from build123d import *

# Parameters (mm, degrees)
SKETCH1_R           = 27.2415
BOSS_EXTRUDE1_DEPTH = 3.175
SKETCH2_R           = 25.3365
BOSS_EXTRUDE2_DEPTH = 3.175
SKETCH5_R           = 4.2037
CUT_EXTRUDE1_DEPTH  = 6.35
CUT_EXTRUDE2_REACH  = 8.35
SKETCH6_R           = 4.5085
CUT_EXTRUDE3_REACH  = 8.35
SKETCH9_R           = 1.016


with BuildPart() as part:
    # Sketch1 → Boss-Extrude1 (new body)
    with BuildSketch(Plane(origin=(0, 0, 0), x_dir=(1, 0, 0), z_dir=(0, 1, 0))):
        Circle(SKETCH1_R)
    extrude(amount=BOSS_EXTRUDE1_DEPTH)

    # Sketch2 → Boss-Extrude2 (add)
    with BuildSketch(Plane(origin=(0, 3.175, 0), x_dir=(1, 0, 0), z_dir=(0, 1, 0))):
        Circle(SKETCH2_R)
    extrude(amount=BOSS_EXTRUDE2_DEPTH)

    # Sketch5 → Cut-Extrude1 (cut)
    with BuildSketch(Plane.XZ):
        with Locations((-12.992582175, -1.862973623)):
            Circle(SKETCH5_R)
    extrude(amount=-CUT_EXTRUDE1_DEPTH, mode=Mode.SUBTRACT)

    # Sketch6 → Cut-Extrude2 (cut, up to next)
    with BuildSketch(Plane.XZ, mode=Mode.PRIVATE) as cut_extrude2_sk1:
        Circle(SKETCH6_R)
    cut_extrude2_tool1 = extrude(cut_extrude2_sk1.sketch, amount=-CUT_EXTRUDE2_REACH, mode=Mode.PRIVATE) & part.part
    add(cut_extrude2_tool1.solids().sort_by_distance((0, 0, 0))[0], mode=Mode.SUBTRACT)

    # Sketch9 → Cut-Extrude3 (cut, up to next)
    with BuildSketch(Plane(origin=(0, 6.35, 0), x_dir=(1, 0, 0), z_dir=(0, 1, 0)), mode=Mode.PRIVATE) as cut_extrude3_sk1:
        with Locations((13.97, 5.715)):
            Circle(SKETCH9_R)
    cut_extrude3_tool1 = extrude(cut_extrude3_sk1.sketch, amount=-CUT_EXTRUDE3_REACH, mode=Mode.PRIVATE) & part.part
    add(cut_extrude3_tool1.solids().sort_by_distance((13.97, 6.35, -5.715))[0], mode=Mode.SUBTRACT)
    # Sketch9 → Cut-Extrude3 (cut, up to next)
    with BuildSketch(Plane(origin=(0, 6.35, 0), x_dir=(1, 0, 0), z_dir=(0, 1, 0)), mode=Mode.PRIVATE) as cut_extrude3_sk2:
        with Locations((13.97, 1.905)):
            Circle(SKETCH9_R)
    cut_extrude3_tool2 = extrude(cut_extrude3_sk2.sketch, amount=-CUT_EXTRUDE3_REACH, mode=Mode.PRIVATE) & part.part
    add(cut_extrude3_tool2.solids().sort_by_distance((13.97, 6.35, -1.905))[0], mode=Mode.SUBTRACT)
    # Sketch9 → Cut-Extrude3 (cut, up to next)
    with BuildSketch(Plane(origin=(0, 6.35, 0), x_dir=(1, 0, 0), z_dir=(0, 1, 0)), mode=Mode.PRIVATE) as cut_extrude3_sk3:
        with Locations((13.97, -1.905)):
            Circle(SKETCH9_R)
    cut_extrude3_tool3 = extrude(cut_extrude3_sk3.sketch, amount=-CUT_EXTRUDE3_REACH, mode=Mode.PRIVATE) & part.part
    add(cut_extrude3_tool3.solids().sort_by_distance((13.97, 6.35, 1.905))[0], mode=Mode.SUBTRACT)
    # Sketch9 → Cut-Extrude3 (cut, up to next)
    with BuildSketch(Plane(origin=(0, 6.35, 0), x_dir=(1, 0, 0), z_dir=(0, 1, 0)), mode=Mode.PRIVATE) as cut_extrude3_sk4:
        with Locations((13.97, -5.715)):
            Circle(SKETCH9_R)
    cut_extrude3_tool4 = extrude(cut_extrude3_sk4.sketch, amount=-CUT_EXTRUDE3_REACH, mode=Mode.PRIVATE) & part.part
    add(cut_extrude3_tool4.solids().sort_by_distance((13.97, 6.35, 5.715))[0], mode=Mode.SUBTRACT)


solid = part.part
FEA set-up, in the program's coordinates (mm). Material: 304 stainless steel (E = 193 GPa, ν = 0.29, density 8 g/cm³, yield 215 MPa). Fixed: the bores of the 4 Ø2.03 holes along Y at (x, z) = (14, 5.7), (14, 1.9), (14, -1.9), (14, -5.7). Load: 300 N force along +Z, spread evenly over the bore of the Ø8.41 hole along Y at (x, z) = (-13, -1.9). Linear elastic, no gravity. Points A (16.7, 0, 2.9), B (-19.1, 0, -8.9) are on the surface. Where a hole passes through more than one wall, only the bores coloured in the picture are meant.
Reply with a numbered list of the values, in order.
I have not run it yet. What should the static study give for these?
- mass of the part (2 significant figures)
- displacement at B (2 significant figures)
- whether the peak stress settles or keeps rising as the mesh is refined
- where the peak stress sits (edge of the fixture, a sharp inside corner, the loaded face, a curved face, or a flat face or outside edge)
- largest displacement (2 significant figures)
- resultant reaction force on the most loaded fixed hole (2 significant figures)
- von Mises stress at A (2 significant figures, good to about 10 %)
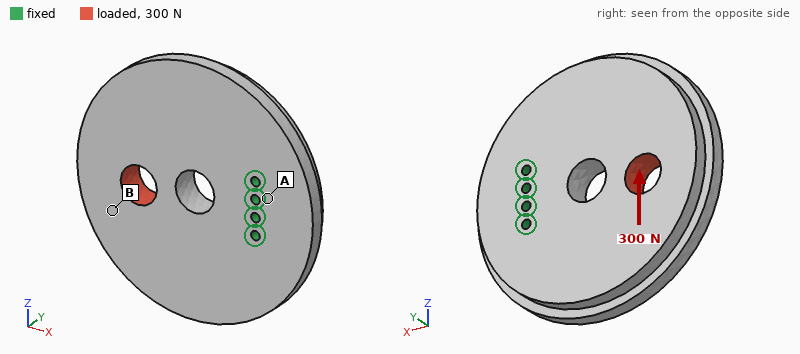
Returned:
1. 100 g
2. 3.5 µm
3. keeps rising
4. edge of the fixture
5. 4.0 µm
6. 580 N
7. 6.7 MPa
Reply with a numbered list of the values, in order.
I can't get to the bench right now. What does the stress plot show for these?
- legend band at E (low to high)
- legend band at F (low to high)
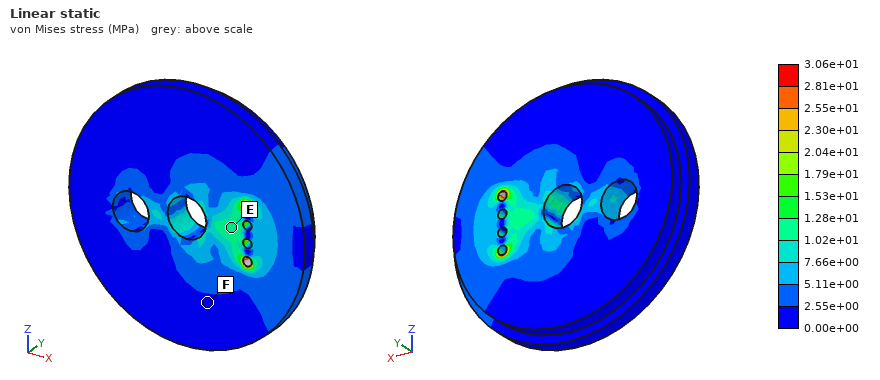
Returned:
1. 1.02e+01 to 1.28e+01 MPa
2. 0.00e+00 to 2.55e+00 MPa
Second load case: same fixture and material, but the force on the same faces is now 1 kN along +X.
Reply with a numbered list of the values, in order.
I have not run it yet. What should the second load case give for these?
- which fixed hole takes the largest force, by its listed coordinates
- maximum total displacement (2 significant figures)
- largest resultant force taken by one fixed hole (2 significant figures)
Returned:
1. (14, -5.7)
2. 1.7 µm
3. 510 N
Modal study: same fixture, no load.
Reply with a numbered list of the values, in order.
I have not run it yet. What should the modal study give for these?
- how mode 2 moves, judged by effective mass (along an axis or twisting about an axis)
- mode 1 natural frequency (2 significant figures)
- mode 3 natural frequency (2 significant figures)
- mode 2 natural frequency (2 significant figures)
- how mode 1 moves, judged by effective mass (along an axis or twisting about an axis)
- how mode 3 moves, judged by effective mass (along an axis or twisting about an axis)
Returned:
1. twisting about X
2. 3100 Hz
3. 6400 Hz
4. 5300 Hz
5. along Y
6. along Z
